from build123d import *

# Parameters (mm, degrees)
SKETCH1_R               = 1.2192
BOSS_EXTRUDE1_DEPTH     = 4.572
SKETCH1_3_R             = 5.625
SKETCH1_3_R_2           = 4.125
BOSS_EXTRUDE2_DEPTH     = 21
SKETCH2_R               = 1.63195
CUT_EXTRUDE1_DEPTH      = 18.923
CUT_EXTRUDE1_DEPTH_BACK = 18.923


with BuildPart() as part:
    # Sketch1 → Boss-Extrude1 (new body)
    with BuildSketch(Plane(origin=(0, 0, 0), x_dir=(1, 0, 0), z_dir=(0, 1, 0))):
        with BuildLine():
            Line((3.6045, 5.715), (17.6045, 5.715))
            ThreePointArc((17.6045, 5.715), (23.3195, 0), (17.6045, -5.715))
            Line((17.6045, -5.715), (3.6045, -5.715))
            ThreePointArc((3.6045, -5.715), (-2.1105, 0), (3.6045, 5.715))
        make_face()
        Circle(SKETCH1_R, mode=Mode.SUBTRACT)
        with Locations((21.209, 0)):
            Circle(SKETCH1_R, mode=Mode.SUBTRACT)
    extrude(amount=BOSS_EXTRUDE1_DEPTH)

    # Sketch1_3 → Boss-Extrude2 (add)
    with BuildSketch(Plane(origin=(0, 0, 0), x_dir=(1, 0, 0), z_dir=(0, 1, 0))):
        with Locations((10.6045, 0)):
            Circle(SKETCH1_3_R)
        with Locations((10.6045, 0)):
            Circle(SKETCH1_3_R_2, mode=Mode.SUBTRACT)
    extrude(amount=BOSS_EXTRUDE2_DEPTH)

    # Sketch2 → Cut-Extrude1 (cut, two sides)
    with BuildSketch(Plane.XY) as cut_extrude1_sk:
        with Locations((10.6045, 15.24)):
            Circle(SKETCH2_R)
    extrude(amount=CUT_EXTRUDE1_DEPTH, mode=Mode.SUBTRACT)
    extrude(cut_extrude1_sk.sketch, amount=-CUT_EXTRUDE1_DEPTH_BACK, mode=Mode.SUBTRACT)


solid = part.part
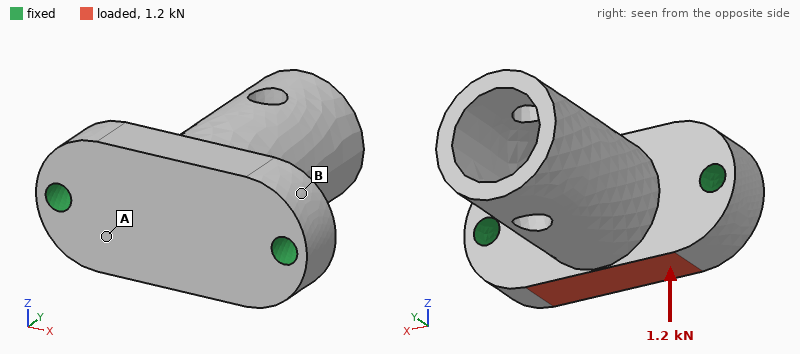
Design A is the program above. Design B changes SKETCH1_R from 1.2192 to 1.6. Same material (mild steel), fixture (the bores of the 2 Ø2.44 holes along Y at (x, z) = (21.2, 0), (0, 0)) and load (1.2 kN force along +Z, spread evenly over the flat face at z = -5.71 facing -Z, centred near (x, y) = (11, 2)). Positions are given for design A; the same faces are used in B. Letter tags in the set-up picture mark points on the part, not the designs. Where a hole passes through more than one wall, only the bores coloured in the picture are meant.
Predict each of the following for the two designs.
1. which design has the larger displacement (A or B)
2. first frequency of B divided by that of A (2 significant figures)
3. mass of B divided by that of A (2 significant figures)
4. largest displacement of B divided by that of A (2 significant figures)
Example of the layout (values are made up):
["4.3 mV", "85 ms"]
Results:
["A", "1.1", "0.98", "0.90"]
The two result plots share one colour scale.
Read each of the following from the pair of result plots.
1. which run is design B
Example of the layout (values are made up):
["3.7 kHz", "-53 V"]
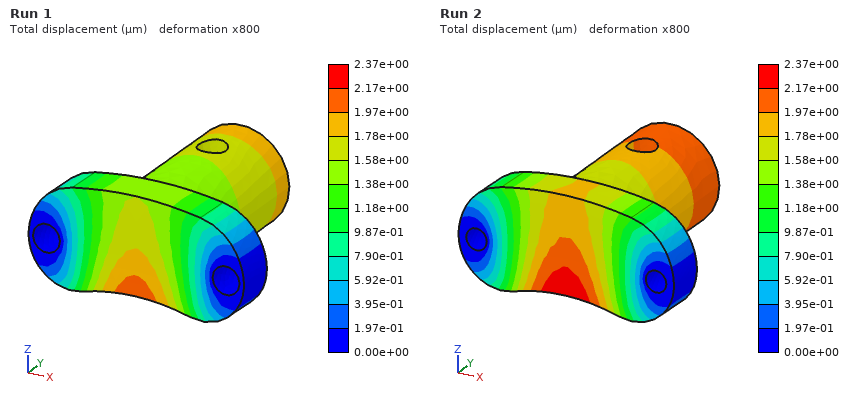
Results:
["Run 1"]
